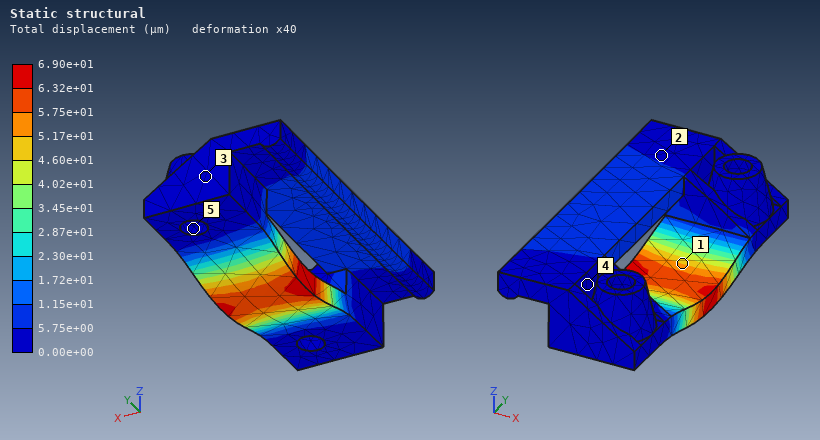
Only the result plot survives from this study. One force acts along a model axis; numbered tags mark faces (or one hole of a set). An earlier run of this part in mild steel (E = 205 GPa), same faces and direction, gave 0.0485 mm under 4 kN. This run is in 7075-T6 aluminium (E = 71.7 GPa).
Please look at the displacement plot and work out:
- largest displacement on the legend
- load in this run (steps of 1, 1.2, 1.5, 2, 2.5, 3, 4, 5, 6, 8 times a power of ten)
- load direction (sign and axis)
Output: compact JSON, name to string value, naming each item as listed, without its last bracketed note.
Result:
{"largest displacement on the legend": "6.90e+01 µm", "load in this run": "2 kN", "load direction": "-Z"}
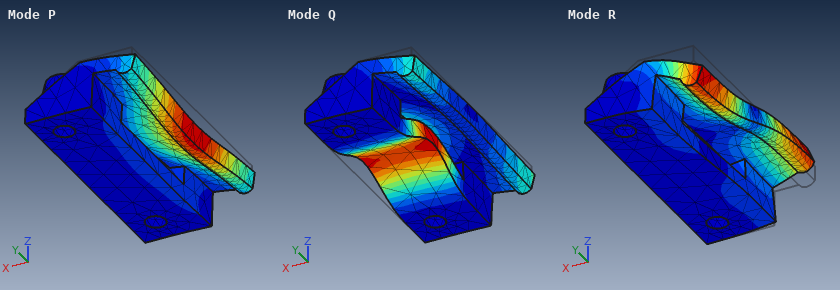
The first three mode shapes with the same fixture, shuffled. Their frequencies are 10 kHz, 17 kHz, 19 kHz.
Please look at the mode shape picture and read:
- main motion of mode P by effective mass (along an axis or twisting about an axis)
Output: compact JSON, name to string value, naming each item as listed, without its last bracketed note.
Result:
{"main motion of mode P by effective mass": "along Z"}
